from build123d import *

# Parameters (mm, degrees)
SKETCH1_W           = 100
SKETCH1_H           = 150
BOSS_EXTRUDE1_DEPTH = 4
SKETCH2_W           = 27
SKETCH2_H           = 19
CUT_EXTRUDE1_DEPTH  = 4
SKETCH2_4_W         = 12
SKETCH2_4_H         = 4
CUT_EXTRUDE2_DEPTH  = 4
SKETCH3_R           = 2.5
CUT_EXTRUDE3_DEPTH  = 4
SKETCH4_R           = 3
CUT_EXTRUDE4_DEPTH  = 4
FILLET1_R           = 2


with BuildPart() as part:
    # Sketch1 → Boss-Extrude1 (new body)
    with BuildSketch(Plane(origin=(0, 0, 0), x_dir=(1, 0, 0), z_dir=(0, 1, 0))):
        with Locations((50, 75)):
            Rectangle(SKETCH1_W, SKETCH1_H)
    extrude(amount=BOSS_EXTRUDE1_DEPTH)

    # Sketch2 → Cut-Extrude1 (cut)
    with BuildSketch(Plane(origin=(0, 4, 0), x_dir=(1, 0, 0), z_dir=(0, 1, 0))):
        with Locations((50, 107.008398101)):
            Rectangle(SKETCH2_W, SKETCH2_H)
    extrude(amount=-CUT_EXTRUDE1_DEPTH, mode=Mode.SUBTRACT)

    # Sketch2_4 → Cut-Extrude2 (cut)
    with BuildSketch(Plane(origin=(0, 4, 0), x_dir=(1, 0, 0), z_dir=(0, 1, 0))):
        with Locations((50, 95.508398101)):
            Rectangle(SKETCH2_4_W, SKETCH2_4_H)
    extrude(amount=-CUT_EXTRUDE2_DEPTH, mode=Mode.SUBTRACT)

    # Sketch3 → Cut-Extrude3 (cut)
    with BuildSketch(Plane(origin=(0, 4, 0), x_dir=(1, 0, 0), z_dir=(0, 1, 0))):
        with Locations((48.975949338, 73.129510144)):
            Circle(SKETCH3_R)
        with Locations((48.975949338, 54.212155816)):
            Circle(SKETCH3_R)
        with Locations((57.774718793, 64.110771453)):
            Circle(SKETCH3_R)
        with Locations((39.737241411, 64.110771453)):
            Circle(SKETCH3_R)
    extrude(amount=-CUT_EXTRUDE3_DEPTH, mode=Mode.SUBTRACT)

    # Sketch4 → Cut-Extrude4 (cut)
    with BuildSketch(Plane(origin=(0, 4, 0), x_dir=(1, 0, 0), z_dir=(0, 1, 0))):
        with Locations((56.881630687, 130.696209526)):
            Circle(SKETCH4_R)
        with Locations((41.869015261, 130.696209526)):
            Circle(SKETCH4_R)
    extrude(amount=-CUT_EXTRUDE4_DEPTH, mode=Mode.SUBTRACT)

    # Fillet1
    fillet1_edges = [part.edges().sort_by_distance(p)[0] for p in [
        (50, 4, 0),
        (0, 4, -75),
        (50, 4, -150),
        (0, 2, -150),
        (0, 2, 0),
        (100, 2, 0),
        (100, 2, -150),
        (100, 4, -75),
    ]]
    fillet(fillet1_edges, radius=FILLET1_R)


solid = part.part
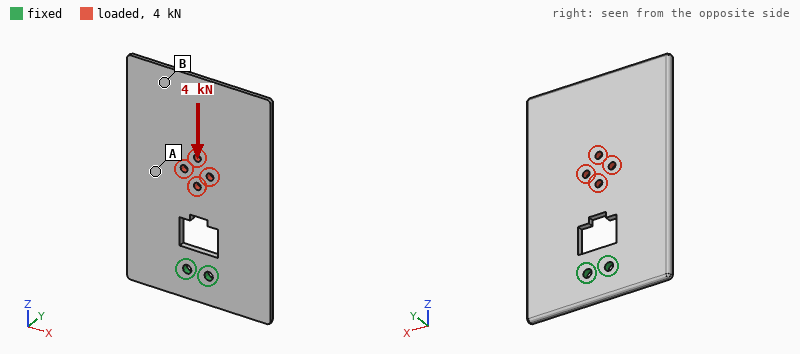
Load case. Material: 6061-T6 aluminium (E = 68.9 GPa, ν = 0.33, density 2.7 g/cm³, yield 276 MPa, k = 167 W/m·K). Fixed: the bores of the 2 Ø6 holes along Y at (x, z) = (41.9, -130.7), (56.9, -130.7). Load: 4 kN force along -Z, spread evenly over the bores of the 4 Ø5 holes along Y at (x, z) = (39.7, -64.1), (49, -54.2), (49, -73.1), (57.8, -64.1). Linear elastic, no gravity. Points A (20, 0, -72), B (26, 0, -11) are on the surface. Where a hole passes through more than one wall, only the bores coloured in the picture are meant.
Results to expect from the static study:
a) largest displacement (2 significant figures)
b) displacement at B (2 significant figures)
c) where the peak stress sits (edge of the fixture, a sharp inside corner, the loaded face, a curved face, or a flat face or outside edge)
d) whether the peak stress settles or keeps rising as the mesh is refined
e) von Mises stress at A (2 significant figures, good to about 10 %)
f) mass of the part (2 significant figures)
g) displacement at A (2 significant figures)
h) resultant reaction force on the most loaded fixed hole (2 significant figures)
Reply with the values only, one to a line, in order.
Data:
35 µm
29 µm
edge of the fixture
keeps rising
9.8 MPa
150 g
26 µm
2.1 kN
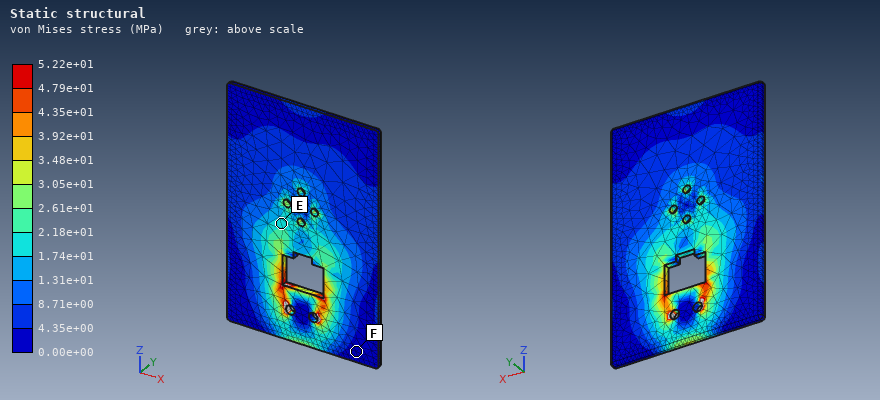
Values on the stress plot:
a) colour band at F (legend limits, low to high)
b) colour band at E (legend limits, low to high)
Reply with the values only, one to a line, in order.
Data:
0.00e+00 to 4.35e+00 MPa
1.74e+01 to 2.18e+01 MPa
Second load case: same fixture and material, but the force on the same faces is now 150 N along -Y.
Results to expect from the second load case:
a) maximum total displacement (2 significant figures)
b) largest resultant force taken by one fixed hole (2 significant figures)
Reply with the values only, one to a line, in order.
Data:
1.6 mm
79 N
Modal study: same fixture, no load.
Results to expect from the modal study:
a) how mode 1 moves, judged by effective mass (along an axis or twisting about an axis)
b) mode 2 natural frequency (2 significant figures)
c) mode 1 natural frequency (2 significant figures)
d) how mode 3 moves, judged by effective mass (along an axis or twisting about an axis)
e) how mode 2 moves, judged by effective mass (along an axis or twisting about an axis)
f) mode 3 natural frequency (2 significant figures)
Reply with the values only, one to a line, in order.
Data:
along Y
450 Hz
150 Hz
along Y
twisting about Z
1000 Hz
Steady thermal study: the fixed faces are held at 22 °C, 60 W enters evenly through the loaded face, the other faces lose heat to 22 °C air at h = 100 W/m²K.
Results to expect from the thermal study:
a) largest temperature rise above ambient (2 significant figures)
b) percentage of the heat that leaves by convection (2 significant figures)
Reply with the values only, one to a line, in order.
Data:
40 K
80 %
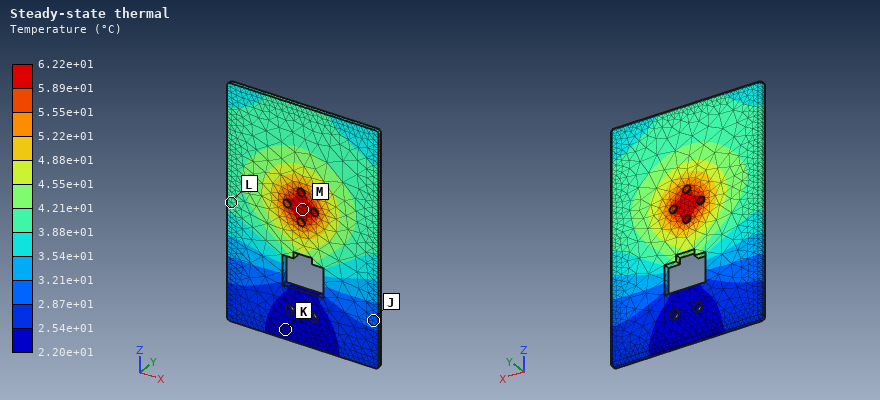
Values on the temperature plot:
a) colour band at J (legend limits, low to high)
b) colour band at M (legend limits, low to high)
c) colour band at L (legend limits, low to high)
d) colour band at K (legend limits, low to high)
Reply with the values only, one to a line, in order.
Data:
2.87e+01 to 3.21e+01 °C
5.89e+01 to 6.22e+01 °C
3.88e+01 to 4.21e+01 °C
2.20e+01 to 2.54e+01 °C
